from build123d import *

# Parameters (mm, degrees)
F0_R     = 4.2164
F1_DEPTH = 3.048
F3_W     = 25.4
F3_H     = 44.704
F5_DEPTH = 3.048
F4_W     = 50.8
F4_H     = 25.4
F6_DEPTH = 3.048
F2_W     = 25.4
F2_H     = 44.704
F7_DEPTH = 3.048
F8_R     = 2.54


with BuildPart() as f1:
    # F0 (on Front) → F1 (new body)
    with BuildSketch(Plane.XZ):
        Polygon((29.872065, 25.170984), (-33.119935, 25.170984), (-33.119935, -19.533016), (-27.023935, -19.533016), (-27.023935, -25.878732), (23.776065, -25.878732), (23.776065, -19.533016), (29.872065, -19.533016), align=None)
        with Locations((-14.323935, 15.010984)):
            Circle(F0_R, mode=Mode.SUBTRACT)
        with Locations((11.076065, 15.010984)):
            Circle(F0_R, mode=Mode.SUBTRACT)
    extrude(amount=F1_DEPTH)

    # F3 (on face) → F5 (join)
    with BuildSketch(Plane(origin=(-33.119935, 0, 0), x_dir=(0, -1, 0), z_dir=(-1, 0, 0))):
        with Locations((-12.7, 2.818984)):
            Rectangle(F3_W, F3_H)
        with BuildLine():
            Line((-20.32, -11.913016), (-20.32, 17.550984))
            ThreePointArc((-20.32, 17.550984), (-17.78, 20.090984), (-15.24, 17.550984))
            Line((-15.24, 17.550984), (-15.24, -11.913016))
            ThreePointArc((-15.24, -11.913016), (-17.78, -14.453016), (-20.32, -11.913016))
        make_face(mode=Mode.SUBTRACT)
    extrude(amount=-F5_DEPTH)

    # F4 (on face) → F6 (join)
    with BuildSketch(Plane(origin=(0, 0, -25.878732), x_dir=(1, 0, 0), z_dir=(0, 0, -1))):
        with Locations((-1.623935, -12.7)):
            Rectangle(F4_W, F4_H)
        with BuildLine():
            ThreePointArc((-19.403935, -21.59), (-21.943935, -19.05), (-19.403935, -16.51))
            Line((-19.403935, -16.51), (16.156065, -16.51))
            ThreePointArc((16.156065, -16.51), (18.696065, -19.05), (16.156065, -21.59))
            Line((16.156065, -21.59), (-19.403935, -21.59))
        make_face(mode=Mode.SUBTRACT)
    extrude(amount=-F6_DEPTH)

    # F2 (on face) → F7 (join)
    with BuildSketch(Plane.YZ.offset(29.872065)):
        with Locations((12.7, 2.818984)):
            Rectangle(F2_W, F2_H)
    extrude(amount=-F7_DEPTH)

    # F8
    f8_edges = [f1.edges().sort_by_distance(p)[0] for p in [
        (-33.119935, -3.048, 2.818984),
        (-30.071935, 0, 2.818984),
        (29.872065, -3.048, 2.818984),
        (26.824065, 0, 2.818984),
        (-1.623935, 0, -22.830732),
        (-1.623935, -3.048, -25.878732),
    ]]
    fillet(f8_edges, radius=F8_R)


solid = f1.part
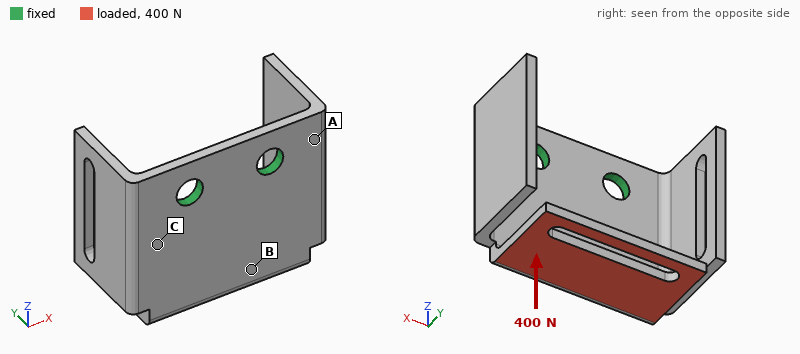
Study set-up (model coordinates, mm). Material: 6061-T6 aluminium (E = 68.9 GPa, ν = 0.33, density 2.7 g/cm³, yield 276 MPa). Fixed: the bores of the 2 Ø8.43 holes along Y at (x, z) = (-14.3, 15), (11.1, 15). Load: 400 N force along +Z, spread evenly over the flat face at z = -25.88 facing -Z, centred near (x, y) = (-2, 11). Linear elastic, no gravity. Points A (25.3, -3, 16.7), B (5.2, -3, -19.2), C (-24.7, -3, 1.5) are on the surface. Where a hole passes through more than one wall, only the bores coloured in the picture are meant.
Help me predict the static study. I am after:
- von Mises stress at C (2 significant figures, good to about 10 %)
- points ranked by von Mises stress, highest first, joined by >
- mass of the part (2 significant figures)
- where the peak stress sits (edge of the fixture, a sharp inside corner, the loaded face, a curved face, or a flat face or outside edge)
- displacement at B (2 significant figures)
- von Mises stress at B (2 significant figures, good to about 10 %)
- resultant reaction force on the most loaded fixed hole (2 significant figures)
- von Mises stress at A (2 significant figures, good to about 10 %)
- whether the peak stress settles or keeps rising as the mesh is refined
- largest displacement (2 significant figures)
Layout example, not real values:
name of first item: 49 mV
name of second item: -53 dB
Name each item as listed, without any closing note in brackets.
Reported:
von Mises stress at C: 9.2 MPa
points ranked by von Mises stress, highest first, joined by >: B > A > C
mass of the part: 51 g
where the peak stress sits: a sharp inside corner
displacement at B: 0.12 mm
von Mises stress at B: 44 MPa
resultant reaction force on the most loaded fixed hole: 200 N
von Mises stress at A: 24 MPa
whether the peak stress settles or keeps rising as the mesh is refined: keeps rising
largest displacement: 0.47 mm
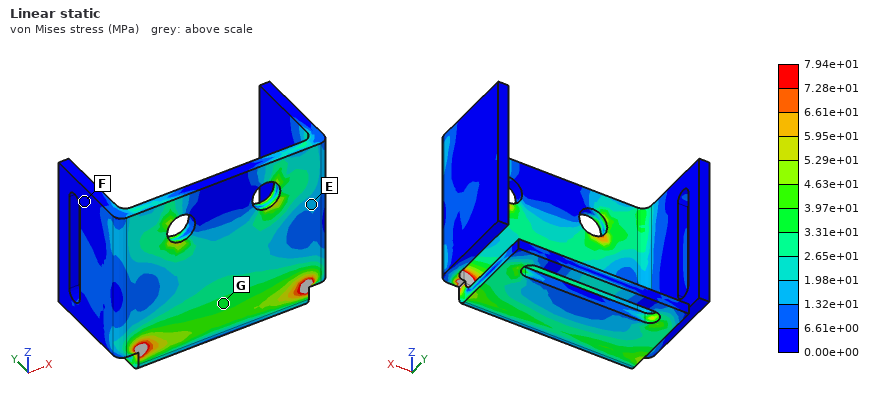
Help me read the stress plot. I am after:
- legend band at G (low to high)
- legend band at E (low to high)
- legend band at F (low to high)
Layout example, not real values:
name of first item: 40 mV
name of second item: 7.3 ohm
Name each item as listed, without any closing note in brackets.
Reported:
legend band at G: 3.31e+01 to 3.97e+01 MPa
legend band at E: 1.32e+01 to 1.98e+01 MPa
legend band at F: 0.00e+00 to 6.61e+00 MPa
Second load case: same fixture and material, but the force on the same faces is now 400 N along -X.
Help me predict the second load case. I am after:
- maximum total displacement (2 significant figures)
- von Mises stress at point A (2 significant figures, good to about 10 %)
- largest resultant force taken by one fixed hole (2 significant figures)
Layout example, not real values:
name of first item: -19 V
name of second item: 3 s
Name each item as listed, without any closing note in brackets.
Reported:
maximum total displacement: 0.20 mm
von Mises stress at point A: 28 MPa
largest resultant force taken by one fixed hole: 540 N
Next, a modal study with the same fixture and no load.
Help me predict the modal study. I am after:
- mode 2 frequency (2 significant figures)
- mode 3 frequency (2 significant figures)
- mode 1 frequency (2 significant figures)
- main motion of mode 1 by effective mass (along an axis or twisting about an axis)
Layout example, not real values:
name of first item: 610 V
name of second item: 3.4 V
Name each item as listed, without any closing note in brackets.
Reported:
mode 2 frequency: 1400 Hz
mode 3 frequency: 2100 Hz
mode 1 frequency: 1100 Hz
main motion of mode 1 by effective mass: along Y
